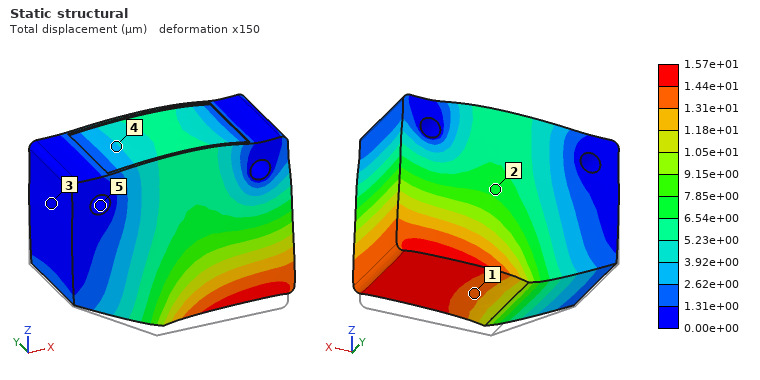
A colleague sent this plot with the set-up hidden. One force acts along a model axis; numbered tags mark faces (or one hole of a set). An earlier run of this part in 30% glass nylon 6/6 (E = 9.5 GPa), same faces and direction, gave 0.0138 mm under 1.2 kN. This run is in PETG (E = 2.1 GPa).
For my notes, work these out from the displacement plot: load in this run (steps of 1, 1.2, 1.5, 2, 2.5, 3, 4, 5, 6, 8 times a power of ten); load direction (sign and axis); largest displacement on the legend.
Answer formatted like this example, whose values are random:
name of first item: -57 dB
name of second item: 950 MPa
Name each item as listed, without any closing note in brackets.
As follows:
load in this run: 300 N
load direction: +Z
largest displacement on the legend: 1.57e+01 µm
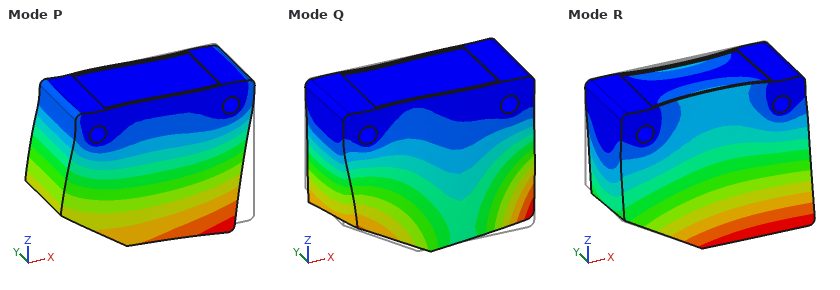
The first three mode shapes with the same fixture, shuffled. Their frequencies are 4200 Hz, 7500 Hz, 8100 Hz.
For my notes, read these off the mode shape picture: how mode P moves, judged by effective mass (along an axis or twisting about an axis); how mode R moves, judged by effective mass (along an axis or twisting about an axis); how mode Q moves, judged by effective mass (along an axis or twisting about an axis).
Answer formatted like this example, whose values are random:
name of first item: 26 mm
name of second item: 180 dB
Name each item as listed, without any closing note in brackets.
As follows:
how mode P moves, judged by effective mass: along X
how mode R moves, judged by effective mass: along Y
how mode Q moves, judged by effective mass: twisting about Z
